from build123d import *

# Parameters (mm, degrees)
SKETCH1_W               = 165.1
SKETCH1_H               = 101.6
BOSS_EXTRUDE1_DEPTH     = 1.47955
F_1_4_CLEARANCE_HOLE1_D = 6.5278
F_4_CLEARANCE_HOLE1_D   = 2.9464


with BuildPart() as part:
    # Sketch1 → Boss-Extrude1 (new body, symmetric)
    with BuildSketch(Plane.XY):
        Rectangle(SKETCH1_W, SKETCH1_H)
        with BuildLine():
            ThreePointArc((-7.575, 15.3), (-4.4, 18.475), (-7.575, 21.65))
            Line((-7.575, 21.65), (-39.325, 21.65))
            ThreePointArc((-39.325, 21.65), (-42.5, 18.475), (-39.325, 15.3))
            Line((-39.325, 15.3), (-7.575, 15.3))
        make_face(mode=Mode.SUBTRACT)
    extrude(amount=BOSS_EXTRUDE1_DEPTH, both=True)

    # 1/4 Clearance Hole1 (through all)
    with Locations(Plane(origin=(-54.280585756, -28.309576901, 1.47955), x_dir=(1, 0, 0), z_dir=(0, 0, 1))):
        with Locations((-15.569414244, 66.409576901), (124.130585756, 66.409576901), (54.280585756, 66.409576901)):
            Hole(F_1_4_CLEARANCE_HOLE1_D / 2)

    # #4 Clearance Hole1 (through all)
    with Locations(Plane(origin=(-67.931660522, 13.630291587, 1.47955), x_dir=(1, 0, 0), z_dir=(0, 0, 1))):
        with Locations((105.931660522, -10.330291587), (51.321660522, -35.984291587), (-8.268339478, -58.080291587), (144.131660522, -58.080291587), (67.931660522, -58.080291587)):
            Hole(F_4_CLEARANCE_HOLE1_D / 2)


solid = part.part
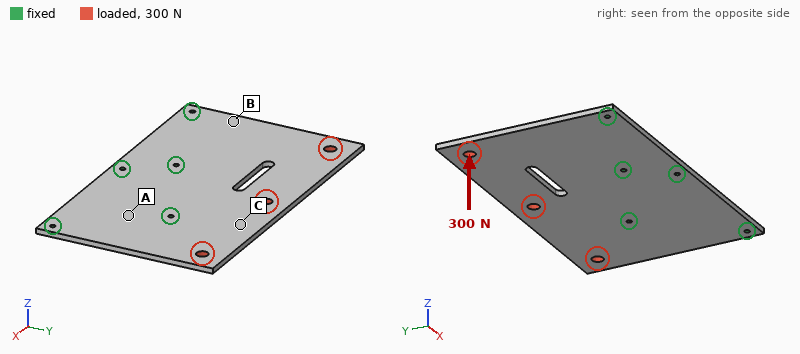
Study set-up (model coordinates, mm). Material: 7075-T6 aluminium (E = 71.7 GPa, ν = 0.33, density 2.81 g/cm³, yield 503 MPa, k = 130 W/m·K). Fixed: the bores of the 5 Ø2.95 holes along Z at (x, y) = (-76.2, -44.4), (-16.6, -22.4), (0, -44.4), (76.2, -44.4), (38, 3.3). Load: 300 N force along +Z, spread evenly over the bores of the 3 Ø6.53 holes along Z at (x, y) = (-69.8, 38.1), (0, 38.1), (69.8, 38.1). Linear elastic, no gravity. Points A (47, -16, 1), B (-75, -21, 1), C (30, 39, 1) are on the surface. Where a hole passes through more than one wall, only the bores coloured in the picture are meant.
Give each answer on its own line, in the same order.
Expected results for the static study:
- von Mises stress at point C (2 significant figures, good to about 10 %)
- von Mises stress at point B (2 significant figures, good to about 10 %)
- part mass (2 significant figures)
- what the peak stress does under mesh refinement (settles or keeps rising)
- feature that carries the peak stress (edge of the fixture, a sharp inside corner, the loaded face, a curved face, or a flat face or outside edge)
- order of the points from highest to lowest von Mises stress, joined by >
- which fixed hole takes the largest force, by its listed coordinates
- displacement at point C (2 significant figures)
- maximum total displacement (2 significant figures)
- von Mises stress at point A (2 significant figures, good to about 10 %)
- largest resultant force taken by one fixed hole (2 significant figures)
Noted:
30 MPa
45 MPa
140 g
keeps rising
edge of the fixture
B > C > A
(38, 3.3)
0.37 mm
1.8 mm
12 MPa
250 N
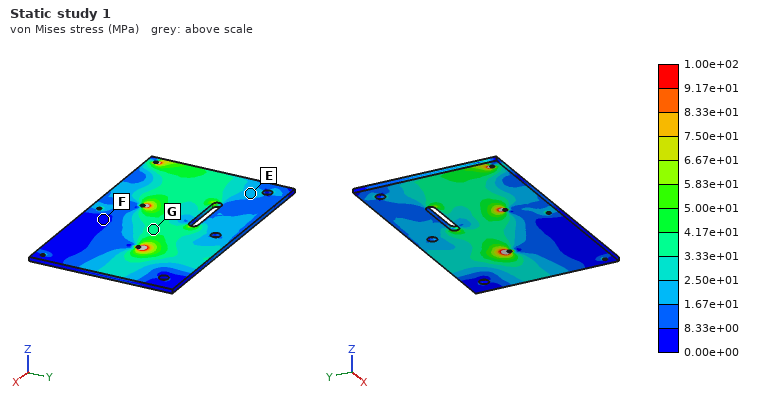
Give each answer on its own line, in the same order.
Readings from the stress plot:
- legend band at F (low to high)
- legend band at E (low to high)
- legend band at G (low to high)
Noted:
0.00e+00 to 8.33e+00 MPa
1.67e+01 to 2.50e+01 MPa
3.33e+01 to 4.17e+01 MPa
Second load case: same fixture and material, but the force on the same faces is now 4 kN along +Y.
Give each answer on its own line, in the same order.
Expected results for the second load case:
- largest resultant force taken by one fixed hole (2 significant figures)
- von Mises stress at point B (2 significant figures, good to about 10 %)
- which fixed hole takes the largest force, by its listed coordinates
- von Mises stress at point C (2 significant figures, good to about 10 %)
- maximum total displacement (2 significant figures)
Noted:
1.2 kN
15 MPa
(38, 3.3)
5.7 MPa
21 µm
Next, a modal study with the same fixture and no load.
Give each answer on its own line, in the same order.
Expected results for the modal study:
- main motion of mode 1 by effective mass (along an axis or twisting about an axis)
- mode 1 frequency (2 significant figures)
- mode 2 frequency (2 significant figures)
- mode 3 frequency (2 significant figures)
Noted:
along Z
420 Hz
840 Hz
1000 Hz
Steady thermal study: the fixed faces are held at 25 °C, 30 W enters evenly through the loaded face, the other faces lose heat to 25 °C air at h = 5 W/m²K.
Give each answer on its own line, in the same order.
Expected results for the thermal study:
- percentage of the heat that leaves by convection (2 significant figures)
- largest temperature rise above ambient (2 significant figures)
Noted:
9.2 %
46 K
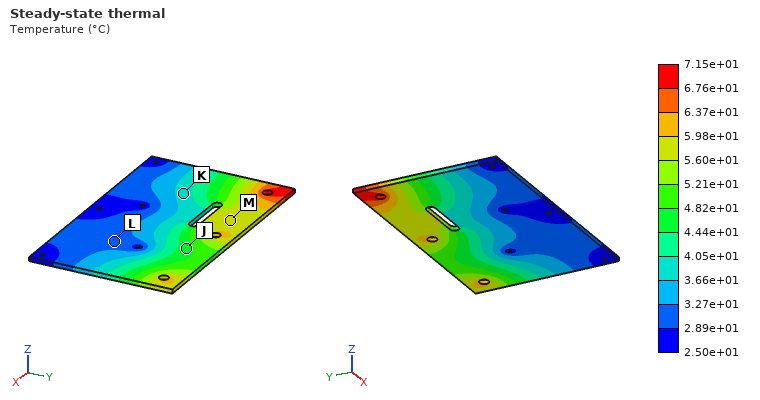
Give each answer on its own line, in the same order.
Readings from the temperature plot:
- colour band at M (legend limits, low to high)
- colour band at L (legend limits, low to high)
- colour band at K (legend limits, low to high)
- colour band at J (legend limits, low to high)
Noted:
5.60e+01 to 5.98e+01 °C
2.89e+01 to 3.27e+01 °C
3.66e+01 to 4.05e+01 °C
4.44e+01 to 4.82e+01 °C
